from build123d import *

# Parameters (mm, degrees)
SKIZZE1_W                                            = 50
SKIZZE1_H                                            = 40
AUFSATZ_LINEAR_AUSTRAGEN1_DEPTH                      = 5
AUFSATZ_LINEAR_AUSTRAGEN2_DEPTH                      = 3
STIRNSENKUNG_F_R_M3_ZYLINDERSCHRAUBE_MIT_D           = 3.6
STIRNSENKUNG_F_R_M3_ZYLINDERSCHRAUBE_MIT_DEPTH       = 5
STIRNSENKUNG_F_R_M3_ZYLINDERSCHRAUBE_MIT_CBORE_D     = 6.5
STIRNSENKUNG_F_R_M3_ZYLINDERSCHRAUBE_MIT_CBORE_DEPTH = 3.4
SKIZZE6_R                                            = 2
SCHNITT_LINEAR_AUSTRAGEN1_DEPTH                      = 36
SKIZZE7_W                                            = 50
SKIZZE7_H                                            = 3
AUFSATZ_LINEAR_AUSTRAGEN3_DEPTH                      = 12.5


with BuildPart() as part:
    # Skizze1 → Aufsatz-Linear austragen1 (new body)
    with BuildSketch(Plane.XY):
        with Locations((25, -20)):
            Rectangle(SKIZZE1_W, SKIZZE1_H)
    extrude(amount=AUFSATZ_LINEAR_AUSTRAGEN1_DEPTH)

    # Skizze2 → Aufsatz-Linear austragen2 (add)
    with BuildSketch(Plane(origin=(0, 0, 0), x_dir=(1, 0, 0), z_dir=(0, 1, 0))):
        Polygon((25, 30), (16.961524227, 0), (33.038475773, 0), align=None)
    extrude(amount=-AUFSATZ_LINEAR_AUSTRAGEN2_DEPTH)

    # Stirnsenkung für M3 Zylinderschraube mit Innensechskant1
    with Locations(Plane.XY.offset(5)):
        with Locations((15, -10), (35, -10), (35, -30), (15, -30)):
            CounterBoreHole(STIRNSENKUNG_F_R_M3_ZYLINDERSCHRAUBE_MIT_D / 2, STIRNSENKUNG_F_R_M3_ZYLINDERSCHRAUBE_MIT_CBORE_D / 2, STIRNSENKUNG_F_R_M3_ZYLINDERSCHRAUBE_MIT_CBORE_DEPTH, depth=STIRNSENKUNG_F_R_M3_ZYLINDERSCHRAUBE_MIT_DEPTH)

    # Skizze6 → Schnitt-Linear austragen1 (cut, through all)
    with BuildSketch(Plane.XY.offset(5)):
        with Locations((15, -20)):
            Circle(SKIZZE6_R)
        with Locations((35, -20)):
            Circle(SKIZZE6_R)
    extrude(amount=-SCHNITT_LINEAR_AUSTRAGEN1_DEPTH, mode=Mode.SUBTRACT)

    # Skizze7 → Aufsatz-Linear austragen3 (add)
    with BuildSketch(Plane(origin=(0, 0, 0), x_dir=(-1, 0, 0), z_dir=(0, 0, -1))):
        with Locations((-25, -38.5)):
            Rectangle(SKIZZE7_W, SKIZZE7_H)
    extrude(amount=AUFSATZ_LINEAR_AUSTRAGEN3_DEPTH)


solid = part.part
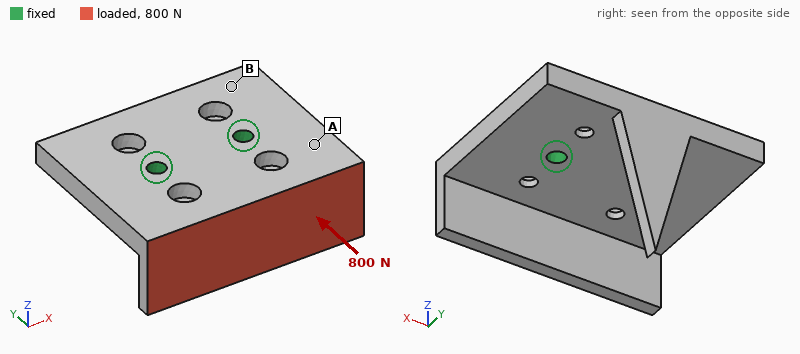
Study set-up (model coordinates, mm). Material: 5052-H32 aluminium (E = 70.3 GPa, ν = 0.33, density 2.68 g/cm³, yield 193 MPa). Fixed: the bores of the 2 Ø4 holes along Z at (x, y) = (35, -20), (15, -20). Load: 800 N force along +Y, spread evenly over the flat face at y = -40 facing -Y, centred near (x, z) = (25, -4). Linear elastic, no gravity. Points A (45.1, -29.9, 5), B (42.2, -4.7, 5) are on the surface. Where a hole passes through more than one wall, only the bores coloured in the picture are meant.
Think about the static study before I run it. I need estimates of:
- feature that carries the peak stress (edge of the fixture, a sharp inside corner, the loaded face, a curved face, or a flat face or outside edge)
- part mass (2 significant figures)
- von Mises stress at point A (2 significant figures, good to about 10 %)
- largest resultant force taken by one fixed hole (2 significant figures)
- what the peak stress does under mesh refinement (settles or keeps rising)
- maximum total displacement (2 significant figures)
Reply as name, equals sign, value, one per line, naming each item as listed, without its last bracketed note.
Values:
feature that carries the peak stress = edge of the fixture
part mass = 32 g
von Mises stress at point A = 22 MPa
largest resultant force taken by one fixed hole = 400 N
what the peak stress does under mesh refinement = keeps rising
maximum total displacement = 76 µm
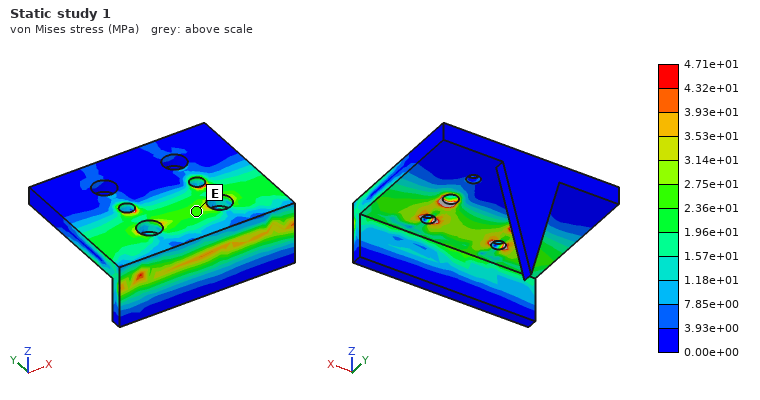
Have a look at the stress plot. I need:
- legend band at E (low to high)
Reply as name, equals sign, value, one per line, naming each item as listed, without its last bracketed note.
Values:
legend band at E = 2.36e+01 to 2.75e+01 MPa
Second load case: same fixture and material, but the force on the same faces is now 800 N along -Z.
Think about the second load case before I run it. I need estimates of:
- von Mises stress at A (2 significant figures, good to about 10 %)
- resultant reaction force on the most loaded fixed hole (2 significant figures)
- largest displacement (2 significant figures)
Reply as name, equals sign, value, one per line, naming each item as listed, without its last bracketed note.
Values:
von Mises stress at A = 38 MPa
resultant reaction force on the most loaded fixed hole = 400 N
largest displacement = 0.12 mm
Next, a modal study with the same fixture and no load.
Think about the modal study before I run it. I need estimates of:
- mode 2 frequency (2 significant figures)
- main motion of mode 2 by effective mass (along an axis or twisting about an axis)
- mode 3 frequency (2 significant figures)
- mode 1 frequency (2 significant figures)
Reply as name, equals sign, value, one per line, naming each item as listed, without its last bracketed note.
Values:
mode 2 frequency = 5100 Hz
main motion of mode 2 by effective mass = along Z
mode 3 frequency = 6400 Hz
mode 1 frequency = 4300 Hz
